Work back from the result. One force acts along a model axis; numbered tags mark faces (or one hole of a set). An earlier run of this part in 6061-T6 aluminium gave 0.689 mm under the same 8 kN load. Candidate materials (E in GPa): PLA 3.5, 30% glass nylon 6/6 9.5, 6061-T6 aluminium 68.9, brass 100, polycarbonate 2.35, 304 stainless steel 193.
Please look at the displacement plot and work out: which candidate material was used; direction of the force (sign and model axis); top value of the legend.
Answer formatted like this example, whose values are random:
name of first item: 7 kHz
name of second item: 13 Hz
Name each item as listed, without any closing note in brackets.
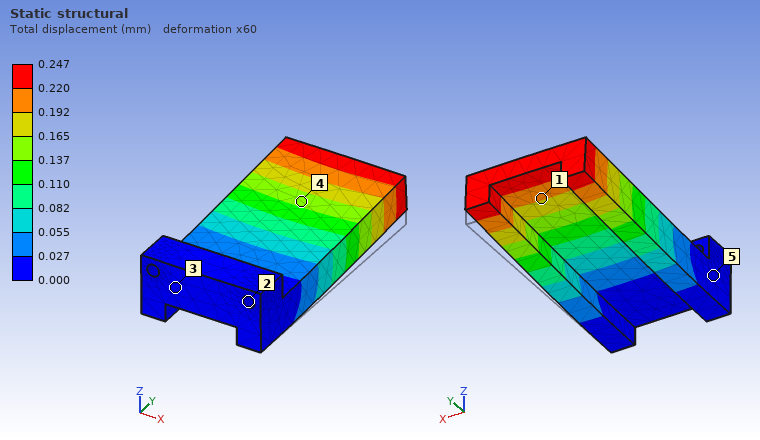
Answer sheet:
which candidate material was used: 304 stainless steel
direction of the force: +Z
top value of the legend: 0.247 mm
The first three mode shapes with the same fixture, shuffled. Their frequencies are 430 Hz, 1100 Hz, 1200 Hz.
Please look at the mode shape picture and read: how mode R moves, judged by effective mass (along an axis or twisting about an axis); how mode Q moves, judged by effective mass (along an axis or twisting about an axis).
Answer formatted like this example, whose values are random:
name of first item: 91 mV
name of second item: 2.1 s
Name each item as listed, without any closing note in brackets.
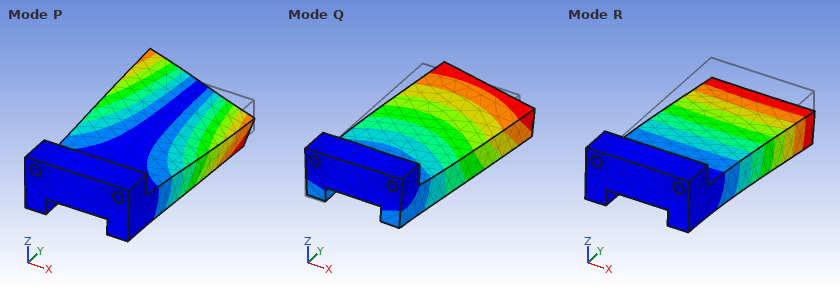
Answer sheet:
how mode R moves, judged by effective mass: along Z
how mode Q moves, judged by effective mass: along X
